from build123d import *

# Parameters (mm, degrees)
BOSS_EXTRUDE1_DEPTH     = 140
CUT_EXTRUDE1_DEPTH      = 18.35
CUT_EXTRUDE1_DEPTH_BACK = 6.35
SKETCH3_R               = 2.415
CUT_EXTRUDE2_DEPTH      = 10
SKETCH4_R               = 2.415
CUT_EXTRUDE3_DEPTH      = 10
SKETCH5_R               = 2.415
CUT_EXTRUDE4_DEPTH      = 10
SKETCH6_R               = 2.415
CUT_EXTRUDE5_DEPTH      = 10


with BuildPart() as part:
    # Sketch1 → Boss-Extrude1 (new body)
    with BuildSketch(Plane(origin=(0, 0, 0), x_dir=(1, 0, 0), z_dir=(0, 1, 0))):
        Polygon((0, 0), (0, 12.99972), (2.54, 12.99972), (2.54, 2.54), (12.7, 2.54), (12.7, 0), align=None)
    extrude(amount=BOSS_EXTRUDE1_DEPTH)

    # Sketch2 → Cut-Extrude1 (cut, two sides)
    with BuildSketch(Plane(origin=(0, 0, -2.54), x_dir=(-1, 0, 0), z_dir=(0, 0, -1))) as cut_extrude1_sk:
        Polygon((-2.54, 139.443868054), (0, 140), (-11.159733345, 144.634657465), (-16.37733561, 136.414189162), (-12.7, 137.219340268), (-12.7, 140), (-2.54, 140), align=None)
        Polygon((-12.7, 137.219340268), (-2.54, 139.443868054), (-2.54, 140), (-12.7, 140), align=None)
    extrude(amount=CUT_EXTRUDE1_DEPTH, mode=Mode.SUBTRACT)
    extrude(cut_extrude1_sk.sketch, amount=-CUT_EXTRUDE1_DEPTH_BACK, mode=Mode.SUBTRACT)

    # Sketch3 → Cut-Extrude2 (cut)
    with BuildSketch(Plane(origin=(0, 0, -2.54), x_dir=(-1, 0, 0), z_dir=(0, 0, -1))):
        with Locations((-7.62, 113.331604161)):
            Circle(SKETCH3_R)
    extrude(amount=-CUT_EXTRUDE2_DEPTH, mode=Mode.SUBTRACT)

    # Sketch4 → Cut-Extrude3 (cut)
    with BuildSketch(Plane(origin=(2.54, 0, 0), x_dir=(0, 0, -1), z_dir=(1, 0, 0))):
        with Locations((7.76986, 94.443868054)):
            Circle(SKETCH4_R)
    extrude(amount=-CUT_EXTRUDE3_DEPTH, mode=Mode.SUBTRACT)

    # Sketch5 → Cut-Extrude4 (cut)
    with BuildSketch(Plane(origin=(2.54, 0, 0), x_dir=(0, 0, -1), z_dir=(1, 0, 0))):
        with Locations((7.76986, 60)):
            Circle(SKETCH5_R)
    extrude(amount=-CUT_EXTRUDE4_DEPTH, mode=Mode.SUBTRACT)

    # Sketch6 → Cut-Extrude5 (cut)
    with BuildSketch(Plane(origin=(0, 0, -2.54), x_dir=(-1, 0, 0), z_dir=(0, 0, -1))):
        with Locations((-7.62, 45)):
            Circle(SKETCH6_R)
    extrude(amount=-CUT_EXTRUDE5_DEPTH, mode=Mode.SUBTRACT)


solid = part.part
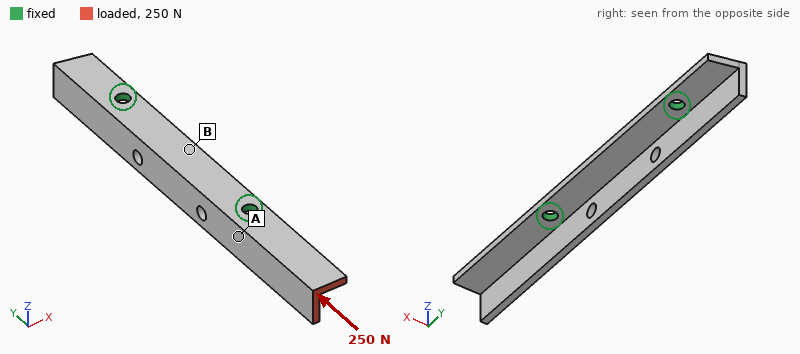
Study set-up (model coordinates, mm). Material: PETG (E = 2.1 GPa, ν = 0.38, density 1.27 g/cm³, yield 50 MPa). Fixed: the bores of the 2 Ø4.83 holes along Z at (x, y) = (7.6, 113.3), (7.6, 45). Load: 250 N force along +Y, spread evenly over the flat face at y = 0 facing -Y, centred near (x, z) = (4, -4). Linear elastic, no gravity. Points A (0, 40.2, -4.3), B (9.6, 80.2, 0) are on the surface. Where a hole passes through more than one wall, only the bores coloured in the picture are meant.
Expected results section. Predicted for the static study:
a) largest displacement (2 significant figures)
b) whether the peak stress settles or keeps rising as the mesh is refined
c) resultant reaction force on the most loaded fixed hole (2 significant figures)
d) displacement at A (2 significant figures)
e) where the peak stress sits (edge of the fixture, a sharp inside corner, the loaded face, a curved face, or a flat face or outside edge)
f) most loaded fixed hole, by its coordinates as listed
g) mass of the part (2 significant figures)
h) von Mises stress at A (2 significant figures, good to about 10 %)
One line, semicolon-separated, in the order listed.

0.33 mm; keeps rising; 200 N; 0.063 mm; edge of the fixture; (7.6, 45); 10 g; 3.9 MPa
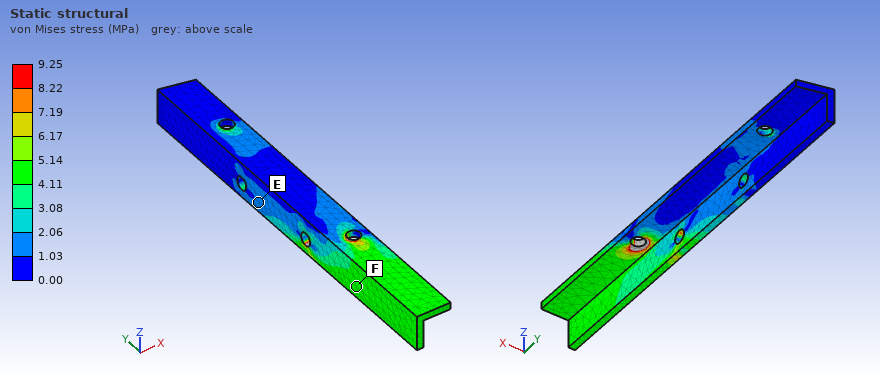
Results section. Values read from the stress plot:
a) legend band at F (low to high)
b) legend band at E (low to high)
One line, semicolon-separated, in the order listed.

4.11 to 5.14 MPa; 1.03 to 2.06 MPa
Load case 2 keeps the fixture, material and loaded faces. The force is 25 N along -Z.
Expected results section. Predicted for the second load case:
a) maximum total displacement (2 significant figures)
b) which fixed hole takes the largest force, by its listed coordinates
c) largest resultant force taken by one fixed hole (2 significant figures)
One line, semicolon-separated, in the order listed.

1.4 mm; (7.6, 45); 53 N
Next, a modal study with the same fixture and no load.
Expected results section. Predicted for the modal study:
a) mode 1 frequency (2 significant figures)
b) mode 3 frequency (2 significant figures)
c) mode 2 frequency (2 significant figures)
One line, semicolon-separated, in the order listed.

660 Hz; 1200 Hz; 870 Hz
